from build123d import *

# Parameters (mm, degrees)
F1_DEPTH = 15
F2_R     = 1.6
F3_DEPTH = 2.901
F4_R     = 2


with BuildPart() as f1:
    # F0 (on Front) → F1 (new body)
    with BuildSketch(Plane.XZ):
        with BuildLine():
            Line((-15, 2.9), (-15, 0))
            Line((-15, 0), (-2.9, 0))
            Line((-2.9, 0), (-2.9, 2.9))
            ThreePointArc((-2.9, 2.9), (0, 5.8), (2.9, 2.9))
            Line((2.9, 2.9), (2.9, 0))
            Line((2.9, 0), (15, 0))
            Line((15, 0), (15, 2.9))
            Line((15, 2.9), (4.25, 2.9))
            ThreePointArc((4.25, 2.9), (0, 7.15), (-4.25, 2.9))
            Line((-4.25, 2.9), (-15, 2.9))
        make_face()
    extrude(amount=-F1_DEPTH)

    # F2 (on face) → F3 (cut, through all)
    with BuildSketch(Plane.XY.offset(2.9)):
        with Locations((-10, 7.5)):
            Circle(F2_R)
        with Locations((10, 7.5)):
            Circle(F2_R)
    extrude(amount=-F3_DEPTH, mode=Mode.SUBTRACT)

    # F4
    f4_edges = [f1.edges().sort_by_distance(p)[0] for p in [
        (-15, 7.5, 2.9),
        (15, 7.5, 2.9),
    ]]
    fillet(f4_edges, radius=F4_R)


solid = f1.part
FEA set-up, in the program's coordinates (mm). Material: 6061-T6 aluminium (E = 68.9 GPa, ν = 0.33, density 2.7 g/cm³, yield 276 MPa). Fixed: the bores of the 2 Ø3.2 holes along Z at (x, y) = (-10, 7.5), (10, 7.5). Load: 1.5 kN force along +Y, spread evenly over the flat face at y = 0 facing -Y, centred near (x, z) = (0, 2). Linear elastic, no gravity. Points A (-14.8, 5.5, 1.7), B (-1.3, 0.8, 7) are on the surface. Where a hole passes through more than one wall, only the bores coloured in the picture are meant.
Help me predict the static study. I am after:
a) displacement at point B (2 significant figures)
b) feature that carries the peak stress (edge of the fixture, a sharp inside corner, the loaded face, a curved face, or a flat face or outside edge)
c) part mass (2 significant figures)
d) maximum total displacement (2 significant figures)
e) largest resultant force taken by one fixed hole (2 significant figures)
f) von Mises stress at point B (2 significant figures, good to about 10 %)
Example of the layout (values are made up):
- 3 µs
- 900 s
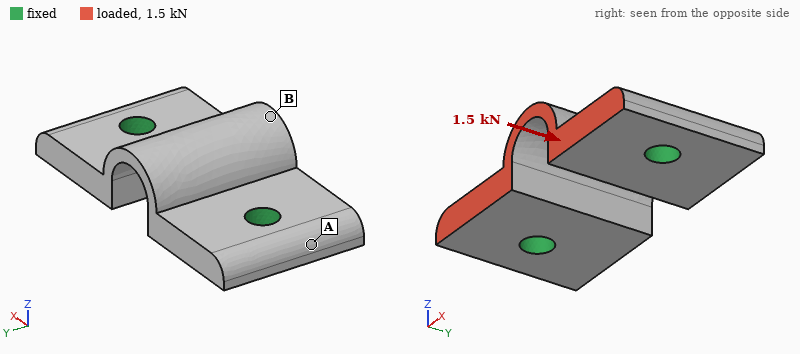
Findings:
- 18 µm
- edge of the fixture
- 3.3 g
- 20 µm
- 750 N
- 27 MPa
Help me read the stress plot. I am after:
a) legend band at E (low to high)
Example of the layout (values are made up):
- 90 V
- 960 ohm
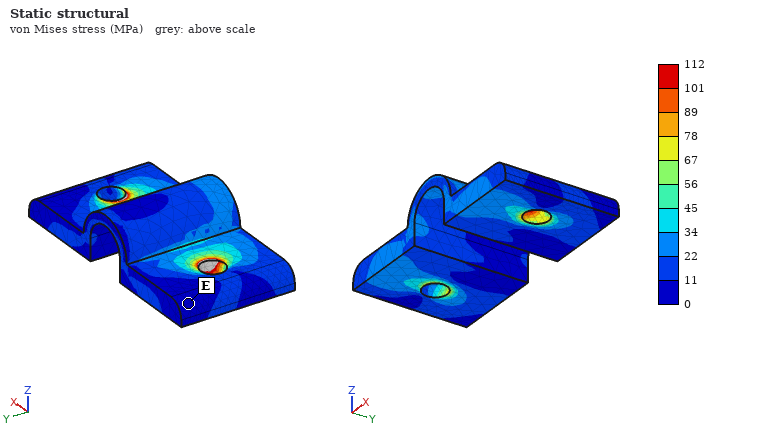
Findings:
- 0 to 11 MPa
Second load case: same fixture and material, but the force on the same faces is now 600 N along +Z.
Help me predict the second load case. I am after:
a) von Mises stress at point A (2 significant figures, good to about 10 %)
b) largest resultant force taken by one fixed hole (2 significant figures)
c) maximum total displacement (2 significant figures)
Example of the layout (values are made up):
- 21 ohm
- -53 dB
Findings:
- 21 MPa
- 300 N
- 31 µm
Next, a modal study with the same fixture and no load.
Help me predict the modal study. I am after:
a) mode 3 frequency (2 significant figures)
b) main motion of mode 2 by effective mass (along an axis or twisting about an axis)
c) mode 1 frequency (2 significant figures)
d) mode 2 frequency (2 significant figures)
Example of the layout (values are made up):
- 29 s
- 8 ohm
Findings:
- 37 kHz
- along Z
- 24 kHz
- 34 kHz
